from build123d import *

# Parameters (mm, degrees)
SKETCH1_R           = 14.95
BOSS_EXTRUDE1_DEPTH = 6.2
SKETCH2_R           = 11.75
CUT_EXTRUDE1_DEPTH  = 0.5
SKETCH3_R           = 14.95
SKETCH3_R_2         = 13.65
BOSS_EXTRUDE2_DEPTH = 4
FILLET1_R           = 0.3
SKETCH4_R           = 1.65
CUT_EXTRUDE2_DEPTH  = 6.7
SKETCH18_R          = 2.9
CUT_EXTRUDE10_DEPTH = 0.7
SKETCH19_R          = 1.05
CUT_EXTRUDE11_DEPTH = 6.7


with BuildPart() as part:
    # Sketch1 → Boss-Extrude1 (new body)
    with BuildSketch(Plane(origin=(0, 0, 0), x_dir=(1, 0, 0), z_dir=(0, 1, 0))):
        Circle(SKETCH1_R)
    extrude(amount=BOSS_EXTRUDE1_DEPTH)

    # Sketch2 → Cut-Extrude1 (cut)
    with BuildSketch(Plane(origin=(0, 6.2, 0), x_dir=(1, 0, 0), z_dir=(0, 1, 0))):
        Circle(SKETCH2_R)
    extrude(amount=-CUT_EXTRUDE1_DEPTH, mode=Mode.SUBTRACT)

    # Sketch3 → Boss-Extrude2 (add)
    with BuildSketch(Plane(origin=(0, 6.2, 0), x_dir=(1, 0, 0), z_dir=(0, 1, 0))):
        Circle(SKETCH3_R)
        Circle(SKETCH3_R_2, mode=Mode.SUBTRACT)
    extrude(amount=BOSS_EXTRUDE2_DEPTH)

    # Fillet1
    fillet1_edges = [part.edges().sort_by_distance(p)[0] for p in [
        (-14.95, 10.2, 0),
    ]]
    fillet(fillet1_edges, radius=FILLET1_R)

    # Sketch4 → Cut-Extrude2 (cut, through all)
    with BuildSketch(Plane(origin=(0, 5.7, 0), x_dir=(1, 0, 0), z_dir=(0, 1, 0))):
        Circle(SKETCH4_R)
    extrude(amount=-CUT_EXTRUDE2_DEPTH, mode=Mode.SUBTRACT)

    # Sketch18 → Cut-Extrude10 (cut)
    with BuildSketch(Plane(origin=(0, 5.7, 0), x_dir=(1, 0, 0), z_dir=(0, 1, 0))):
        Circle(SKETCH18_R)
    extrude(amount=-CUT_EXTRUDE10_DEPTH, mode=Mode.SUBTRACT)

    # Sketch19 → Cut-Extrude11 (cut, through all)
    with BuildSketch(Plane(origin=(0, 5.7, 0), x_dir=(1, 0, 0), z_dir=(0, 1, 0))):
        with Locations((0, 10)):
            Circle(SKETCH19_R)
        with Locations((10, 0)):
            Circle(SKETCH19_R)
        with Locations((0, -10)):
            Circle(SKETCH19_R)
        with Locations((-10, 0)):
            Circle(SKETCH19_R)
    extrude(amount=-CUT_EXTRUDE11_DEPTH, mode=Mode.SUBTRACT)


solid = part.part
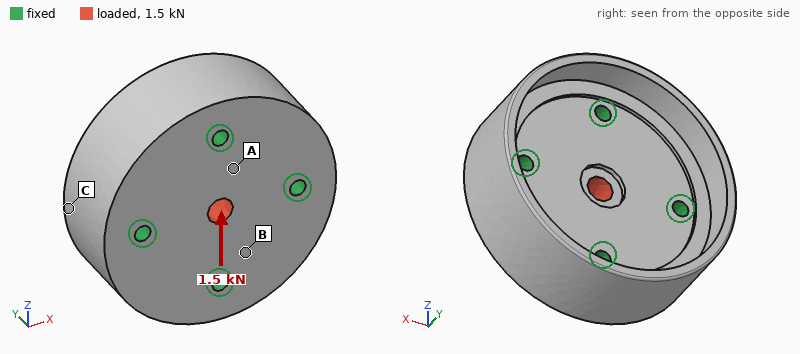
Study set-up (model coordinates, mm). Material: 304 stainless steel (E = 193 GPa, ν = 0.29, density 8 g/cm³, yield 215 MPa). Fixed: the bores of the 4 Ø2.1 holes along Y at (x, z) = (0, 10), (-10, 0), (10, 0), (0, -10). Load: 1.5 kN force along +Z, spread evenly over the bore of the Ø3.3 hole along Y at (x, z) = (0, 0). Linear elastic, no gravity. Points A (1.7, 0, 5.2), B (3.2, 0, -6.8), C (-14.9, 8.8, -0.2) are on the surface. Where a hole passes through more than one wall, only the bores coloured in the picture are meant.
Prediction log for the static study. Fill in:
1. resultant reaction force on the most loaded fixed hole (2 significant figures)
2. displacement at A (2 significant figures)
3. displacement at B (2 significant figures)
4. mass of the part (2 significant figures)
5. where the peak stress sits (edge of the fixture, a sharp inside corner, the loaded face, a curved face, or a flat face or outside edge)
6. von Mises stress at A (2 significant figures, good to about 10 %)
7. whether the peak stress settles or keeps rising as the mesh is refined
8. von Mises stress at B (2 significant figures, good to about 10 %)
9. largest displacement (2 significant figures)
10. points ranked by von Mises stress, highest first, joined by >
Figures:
490 N
0.37 µm
0.28 µm
36 g
a sharp inside corner
16 MPa
keeps rising
8.2 MPa
0.84 µm
A > B > C
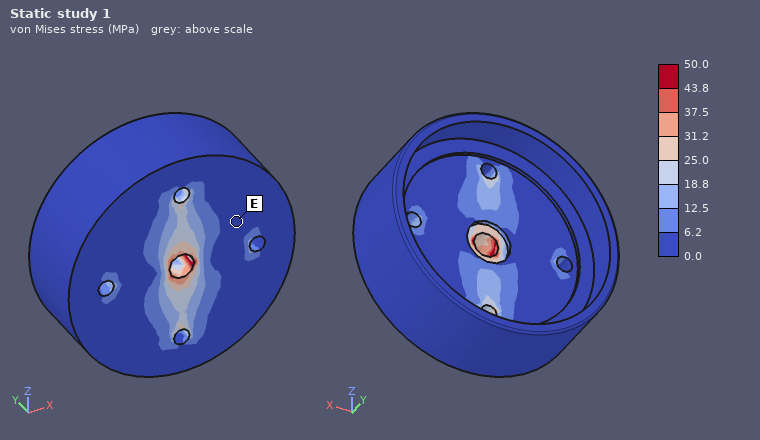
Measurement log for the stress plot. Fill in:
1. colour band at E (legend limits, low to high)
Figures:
0.0 to 6.2 MPa
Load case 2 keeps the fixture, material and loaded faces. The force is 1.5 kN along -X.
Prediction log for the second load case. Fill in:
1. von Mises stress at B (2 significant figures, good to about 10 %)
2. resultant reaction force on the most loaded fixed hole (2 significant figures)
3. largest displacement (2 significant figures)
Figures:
4.4 MPa
490 N
0.84 µm
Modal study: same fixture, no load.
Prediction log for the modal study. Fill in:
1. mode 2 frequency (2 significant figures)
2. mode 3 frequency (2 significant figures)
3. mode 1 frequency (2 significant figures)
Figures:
43 kHz
43 kHz
38 kHz
